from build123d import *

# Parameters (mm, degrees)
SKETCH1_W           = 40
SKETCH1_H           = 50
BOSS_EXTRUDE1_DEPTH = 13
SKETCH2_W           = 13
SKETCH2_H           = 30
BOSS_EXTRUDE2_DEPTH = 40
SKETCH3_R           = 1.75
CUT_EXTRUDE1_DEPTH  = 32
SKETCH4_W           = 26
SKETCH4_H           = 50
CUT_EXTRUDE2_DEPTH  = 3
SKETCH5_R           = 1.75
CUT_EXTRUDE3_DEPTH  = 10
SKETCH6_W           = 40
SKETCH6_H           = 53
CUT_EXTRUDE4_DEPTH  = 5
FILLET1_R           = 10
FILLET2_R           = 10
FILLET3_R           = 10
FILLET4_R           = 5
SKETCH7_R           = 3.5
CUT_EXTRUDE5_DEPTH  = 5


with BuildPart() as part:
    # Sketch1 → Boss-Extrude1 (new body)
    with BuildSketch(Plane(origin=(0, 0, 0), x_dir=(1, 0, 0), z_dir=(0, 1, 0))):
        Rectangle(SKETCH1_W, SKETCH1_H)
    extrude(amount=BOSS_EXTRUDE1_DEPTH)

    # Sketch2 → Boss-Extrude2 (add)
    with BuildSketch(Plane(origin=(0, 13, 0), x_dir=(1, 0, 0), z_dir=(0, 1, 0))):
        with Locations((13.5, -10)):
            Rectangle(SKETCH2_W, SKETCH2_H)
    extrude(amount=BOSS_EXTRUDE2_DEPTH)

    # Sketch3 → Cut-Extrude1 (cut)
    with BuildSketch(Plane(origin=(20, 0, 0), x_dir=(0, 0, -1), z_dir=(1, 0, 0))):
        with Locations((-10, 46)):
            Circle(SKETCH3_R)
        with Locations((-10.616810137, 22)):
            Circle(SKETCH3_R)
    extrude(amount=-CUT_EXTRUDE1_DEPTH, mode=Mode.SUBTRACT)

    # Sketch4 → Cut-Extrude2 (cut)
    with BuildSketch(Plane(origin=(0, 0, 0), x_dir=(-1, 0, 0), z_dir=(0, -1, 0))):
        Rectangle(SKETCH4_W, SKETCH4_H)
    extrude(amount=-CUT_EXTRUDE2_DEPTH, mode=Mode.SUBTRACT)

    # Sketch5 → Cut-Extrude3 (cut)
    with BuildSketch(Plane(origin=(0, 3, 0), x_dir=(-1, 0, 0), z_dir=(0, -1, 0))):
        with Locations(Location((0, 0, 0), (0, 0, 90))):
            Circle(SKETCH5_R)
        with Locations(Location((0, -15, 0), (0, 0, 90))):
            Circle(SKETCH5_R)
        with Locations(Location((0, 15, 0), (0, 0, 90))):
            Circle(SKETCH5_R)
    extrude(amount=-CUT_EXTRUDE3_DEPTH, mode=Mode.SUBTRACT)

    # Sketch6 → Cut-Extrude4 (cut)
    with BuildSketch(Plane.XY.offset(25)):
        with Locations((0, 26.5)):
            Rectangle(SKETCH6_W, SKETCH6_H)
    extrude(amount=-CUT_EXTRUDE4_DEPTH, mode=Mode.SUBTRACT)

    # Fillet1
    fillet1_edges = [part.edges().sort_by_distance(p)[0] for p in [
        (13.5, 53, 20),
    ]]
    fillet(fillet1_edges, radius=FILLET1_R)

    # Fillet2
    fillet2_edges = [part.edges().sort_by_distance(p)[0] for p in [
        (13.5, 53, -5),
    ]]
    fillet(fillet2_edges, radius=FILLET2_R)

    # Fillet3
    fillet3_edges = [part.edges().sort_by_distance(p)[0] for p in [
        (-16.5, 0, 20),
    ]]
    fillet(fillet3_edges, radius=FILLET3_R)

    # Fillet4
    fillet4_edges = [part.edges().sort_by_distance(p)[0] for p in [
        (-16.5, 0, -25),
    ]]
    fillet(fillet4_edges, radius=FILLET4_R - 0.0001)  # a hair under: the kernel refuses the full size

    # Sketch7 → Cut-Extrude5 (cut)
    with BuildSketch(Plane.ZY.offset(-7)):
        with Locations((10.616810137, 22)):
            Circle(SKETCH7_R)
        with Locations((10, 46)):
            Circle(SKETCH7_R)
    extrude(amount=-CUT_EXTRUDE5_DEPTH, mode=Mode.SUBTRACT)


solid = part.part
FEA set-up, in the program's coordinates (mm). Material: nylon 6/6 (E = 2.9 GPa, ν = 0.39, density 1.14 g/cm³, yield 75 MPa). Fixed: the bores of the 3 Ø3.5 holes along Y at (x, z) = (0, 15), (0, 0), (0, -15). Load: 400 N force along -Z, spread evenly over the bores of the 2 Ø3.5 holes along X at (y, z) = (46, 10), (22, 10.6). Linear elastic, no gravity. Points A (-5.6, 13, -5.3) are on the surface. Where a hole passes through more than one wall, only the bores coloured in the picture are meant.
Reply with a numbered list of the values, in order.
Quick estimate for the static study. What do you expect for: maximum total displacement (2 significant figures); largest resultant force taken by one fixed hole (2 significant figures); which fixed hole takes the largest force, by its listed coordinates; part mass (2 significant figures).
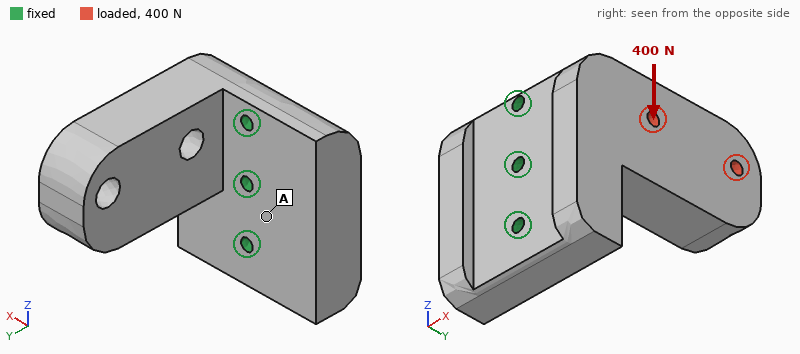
1. 0.35 mm
2. 470 N
3. (0, 15)
4. 35 g
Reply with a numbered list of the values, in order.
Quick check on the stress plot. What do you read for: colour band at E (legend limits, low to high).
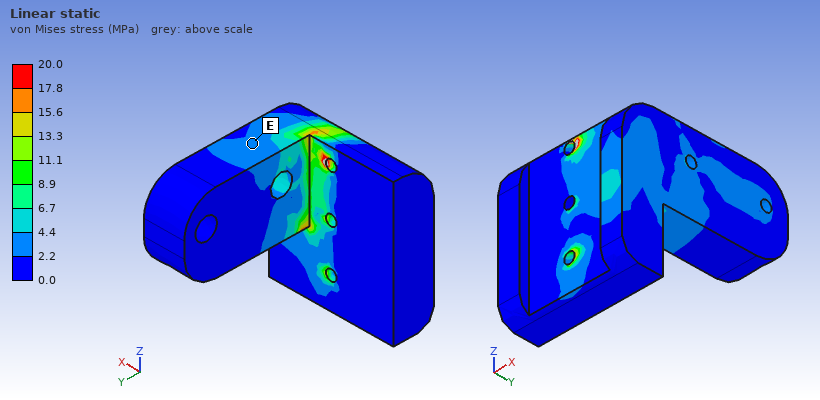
1. 2.2 to 4.4 MPa
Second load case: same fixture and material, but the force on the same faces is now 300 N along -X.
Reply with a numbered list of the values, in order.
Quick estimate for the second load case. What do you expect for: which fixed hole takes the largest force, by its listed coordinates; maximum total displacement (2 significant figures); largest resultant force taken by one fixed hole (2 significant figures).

1. (0, 15)
2. 0.79 mm
3. 180 N
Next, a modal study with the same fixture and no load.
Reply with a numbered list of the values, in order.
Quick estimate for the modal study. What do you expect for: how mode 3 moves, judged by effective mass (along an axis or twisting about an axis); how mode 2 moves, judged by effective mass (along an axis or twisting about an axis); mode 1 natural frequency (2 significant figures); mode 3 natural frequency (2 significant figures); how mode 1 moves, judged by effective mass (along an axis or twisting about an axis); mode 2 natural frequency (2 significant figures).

1. along Y
2. along Z
3. 1100 Hz
4. 3800 Hz
5. along X
6. 1800 Hz
